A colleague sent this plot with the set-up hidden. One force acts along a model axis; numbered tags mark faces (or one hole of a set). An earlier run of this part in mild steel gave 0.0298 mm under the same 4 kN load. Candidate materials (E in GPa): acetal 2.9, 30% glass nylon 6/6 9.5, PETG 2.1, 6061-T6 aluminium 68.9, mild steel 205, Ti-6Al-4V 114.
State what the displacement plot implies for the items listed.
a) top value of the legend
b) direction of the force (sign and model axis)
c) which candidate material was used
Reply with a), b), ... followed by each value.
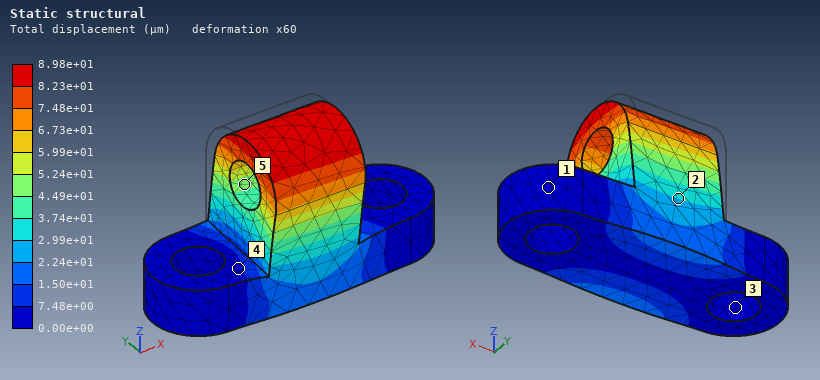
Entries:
a) 8.98e+01 µm
b) -Y
c) 6061-T6 aluminium
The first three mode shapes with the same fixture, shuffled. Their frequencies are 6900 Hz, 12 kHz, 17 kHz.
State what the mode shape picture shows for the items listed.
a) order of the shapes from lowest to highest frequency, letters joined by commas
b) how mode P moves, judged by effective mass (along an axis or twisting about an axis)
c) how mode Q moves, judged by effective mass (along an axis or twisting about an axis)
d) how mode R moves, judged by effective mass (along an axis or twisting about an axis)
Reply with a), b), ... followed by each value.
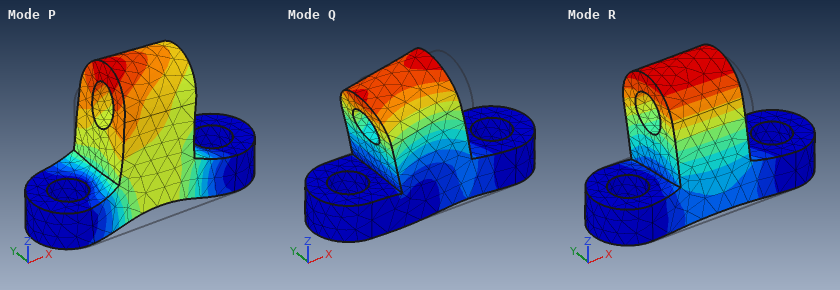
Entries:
a) R, Q, P
b) along Z
c) along X
d) along Y
